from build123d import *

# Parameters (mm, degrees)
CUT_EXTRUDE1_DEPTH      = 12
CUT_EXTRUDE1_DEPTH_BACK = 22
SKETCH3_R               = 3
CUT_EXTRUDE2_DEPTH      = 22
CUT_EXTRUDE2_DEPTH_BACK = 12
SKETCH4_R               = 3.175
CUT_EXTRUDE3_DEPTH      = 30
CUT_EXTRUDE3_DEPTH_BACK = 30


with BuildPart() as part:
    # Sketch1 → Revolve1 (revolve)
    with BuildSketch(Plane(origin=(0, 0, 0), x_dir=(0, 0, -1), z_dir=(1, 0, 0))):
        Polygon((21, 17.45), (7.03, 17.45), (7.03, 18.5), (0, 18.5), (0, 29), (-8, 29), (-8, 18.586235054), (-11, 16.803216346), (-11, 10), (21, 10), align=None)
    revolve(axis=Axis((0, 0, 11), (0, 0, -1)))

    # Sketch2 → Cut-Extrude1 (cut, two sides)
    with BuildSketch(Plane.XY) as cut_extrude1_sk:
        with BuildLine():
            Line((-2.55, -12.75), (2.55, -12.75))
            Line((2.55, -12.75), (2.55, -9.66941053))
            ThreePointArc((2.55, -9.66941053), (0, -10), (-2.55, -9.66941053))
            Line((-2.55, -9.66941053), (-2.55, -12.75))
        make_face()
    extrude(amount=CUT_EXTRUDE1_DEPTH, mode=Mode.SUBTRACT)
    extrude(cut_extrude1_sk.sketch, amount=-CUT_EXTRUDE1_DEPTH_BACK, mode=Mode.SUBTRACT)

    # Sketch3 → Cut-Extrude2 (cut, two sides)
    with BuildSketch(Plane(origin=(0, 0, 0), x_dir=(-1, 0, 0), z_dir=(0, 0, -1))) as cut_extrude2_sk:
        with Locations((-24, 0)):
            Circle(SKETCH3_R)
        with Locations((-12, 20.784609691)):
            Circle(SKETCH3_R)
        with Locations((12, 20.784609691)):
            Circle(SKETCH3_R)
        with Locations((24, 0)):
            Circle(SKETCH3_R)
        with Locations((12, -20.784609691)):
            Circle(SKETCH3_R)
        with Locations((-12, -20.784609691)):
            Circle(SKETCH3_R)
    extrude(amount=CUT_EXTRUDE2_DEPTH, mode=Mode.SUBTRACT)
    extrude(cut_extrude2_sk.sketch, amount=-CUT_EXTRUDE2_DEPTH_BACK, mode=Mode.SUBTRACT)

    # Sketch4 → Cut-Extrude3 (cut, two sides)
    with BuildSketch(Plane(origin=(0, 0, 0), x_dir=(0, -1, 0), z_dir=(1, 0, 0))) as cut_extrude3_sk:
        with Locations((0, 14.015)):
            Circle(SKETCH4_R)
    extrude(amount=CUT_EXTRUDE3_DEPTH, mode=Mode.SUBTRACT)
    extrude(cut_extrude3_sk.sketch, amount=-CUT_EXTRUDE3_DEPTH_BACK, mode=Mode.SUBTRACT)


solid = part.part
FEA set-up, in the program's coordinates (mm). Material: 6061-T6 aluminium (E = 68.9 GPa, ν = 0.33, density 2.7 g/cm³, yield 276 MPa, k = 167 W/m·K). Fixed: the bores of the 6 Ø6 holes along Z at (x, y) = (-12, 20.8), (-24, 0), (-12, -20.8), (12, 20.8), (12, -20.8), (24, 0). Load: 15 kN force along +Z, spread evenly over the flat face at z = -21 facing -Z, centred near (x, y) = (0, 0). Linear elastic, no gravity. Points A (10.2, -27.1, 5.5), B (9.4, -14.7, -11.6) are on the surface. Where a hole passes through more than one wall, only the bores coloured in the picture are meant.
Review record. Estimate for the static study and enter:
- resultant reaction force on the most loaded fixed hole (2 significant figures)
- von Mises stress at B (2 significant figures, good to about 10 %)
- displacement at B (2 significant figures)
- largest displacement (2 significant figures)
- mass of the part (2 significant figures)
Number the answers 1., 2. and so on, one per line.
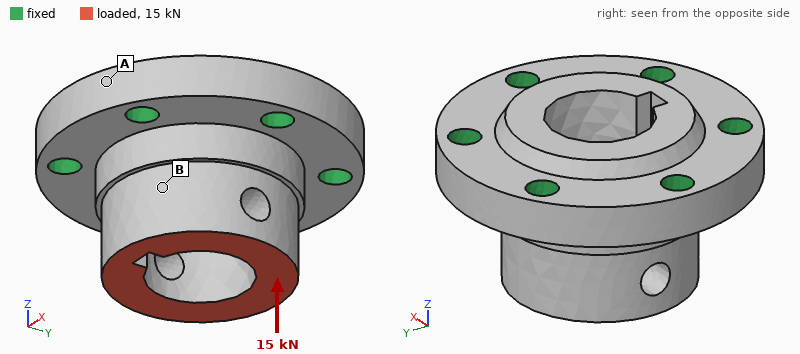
1. 2.7 kN
2. 23 MPa
3. 11 µm
4. 19 µm
5. 88 g
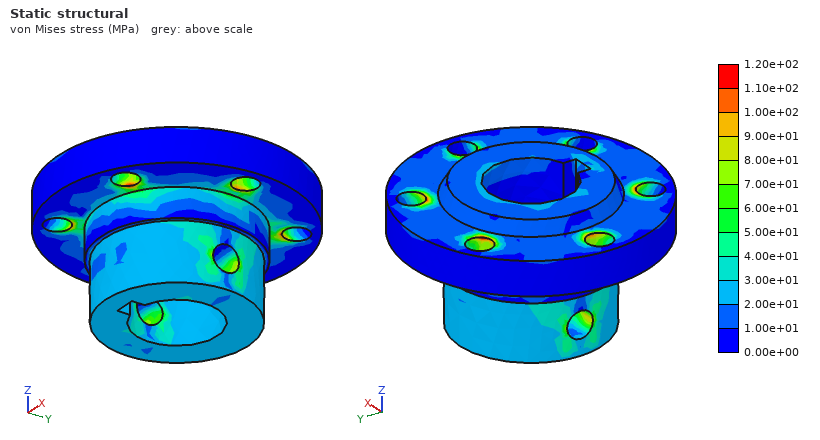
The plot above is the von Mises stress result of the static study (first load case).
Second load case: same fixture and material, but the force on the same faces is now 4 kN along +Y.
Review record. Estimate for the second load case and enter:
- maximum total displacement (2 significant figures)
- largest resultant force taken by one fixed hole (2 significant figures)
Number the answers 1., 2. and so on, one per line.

1. 23 µm
2. 1.6 kN
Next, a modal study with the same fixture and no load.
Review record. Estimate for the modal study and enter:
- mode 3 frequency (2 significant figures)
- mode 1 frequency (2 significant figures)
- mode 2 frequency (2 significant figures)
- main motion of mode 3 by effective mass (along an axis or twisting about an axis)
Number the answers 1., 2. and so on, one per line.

1. 27 kHz
2. 20 kHz
3. 21 kHz
4. along Z
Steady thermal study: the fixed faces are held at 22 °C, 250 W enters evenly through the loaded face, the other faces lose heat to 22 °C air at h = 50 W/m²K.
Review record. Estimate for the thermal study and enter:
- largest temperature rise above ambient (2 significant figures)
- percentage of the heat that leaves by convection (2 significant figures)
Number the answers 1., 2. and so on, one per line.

1. 70 K
2. 3.8 %
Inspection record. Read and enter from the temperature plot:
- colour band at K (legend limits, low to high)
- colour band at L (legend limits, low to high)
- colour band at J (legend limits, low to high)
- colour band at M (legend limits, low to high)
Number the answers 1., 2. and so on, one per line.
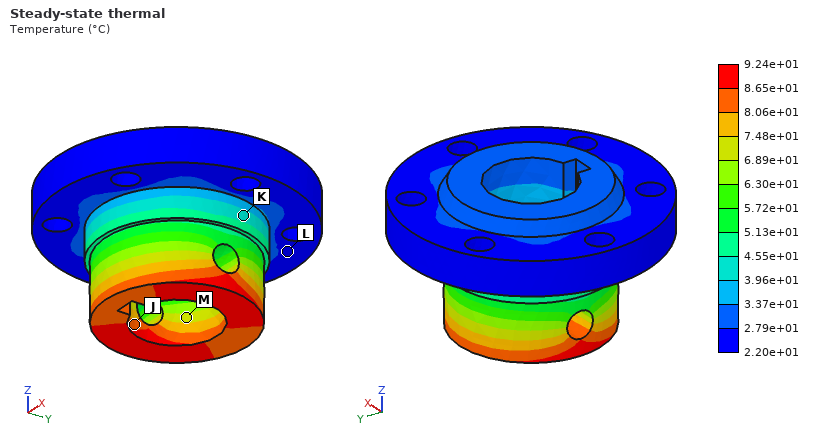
1. 3.96e+01 to 4.55e+01 °C
2. 2.20e+01 to 2.79e+01 °C
3. 8.06e+01 to 8.65e+01 °C
4. 6.89e+01 to 7.48e+01 °C
